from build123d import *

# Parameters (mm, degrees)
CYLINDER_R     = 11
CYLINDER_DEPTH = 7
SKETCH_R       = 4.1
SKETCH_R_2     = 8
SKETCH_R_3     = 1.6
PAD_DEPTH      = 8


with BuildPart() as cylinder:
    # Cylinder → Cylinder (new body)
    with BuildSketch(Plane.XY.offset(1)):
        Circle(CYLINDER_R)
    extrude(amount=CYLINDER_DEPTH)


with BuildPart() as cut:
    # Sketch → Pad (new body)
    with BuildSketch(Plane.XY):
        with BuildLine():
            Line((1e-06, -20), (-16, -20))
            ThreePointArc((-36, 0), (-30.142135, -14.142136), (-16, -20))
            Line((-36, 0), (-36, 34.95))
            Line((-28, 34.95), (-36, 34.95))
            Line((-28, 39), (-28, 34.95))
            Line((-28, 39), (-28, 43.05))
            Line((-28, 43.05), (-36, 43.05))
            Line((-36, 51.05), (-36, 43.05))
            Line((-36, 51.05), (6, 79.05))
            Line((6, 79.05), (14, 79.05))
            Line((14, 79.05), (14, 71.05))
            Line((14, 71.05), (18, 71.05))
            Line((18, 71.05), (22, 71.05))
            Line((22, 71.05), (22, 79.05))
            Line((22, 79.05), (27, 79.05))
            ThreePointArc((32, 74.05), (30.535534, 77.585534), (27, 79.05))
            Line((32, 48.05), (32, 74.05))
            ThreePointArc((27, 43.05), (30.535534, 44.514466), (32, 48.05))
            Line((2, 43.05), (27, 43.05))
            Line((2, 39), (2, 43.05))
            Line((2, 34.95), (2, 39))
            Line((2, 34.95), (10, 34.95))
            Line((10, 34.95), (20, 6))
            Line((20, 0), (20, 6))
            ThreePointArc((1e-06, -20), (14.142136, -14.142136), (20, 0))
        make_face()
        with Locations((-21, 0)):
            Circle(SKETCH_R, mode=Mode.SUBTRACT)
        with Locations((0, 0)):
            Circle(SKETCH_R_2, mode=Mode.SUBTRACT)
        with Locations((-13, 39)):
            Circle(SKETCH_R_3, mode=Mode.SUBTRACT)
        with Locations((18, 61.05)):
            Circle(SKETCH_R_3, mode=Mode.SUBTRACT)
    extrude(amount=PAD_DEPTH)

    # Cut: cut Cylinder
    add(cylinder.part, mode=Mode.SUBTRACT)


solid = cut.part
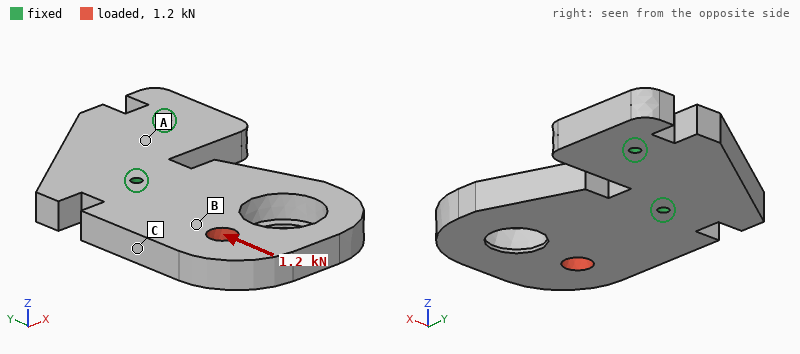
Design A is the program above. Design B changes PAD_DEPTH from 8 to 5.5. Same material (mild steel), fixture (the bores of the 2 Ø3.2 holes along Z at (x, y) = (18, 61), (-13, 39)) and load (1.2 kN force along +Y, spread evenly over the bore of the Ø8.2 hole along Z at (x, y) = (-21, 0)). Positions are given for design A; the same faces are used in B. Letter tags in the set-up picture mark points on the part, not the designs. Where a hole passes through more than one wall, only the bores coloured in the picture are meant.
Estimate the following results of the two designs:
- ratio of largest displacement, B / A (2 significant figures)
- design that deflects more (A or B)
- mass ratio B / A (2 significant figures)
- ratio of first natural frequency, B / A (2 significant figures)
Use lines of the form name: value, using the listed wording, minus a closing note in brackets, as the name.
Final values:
ratio of largest displacement, B / A: 1.5
design that deflects more: B
mass ratio B / A: 0.69
ratio of first natural frequency, B / A: 0.72
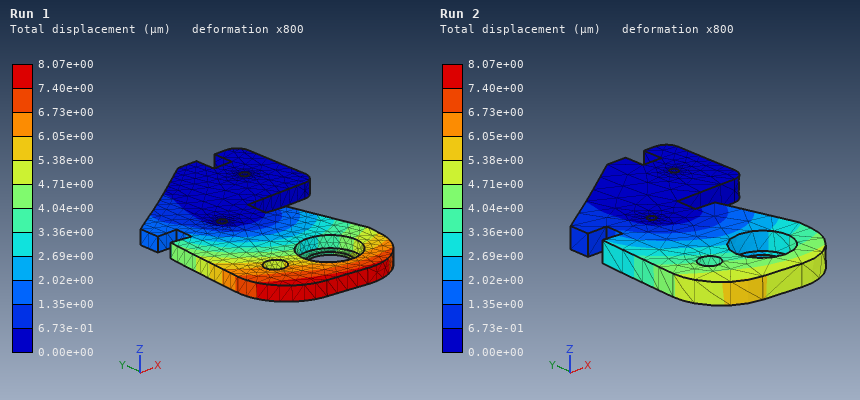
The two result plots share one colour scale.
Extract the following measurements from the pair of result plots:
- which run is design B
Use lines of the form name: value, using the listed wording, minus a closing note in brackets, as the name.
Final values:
which run is design B: Run 1
